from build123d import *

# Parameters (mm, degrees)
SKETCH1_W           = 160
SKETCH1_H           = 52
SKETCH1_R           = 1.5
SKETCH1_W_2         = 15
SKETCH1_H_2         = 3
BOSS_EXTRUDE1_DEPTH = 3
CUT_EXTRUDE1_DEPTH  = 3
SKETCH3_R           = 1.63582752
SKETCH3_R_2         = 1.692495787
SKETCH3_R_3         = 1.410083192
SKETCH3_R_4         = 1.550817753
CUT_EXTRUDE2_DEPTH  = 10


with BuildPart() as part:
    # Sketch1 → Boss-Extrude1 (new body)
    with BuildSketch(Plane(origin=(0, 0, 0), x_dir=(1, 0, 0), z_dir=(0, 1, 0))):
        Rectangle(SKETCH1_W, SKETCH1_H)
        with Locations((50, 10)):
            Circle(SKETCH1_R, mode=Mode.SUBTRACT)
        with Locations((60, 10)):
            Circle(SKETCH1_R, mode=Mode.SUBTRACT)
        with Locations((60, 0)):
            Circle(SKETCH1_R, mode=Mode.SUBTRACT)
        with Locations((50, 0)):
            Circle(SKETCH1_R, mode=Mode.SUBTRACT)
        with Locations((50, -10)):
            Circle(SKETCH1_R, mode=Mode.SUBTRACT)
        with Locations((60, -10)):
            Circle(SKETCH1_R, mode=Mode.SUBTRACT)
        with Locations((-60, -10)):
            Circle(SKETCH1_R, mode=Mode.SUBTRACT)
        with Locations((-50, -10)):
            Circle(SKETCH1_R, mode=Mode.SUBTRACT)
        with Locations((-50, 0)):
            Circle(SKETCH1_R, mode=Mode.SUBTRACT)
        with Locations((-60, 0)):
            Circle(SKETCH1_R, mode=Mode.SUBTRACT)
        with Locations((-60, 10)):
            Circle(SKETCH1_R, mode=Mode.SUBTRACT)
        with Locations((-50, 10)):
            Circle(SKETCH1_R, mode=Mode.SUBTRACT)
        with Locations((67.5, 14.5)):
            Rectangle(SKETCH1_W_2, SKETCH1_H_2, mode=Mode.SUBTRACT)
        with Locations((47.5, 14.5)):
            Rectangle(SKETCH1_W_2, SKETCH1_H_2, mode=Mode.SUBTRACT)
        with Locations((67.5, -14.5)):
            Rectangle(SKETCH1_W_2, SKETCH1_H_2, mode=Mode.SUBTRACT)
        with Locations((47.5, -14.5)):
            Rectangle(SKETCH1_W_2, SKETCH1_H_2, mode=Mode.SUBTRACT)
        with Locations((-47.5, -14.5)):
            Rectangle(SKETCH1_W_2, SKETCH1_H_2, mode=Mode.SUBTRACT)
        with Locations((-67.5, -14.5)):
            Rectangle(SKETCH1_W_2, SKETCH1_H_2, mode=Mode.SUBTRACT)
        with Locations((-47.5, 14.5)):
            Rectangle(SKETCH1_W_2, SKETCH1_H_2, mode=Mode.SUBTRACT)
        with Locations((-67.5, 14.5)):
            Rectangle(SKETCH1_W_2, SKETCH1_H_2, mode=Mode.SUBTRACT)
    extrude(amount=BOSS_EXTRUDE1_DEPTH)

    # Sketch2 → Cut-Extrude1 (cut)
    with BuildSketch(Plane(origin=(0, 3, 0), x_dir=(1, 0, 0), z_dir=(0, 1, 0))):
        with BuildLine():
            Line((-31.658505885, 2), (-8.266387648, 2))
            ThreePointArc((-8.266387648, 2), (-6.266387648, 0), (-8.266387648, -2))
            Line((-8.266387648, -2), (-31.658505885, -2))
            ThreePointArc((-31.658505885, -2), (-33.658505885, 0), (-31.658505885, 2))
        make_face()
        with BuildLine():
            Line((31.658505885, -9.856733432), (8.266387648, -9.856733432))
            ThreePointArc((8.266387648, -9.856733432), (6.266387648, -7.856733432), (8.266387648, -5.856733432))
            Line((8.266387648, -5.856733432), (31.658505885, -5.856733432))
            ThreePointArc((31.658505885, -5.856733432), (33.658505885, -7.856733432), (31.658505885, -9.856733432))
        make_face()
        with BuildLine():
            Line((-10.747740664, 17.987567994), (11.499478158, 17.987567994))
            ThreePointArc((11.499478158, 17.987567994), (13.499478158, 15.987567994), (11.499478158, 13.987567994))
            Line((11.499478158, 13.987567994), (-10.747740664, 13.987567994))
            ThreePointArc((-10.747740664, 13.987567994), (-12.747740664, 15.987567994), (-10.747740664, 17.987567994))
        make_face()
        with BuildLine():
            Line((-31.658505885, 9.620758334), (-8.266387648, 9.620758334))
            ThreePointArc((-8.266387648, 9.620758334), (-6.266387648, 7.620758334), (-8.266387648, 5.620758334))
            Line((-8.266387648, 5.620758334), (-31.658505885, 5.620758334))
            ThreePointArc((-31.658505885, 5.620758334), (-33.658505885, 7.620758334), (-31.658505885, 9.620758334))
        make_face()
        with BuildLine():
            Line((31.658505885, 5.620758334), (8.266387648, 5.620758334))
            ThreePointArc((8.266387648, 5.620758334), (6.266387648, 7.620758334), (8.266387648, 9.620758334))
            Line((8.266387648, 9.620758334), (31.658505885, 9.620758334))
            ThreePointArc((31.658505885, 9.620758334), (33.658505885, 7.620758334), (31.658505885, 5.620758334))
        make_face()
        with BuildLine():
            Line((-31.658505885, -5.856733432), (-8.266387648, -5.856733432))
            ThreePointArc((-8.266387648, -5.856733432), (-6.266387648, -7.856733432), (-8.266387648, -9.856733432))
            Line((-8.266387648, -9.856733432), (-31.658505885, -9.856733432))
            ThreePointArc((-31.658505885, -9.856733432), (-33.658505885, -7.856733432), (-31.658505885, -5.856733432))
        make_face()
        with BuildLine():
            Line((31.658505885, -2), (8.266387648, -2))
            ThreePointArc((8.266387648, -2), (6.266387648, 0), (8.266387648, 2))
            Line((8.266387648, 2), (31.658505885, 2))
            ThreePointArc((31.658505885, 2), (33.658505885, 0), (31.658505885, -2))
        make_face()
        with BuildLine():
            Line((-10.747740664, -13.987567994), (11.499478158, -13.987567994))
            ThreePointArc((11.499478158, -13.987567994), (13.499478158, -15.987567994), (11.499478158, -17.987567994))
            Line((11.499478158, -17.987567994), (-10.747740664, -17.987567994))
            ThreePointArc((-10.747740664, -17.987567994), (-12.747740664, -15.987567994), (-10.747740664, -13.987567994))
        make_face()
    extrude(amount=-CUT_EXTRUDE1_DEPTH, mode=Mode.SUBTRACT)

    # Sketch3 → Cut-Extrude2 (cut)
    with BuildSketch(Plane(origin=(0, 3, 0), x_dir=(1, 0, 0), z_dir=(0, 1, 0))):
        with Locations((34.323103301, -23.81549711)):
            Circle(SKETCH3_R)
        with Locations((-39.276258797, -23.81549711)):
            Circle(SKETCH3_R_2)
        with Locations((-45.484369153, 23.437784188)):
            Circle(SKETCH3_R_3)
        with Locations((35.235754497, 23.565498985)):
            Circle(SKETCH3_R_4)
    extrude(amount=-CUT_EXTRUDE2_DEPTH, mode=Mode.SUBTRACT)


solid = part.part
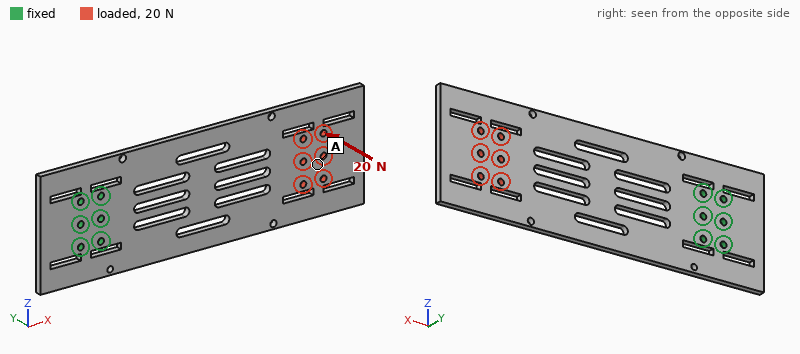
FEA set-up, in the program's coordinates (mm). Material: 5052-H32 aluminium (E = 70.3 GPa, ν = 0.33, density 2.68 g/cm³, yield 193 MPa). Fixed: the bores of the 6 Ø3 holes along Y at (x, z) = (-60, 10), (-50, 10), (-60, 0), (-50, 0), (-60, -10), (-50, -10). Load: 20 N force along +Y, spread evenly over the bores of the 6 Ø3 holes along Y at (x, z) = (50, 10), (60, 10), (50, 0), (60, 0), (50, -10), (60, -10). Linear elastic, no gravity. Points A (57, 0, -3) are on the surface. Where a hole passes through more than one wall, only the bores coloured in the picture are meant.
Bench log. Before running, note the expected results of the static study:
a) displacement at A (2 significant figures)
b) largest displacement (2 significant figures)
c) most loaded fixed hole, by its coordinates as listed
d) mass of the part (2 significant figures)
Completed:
1.2 mm
1.6 mm
(-50, 0)
56 g
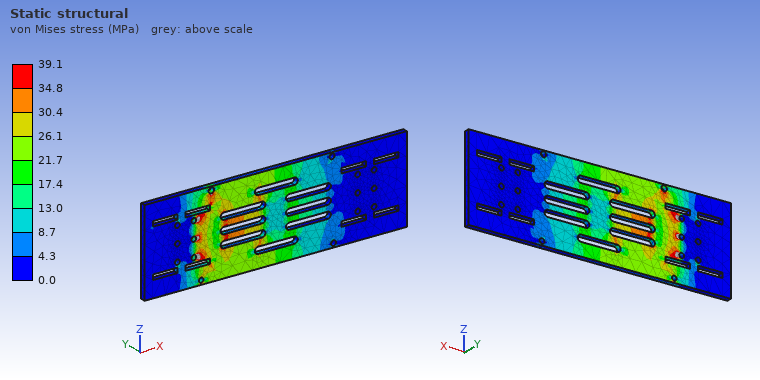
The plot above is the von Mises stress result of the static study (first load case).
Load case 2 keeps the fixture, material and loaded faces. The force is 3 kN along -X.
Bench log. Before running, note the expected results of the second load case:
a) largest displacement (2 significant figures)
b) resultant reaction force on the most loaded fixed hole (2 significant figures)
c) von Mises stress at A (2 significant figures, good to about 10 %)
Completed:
50 µm
820 N
12 MPa
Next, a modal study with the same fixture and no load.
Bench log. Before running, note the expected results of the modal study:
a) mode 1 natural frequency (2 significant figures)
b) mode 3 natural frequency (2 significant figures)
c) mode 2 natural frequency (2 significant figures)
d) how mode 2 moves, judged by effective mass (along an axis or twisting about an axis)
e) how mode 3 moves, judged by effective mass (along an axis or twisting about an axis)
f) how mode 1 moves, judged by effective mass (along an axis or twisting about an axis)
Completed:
140 Hz
880 Hz
610 Hz
twisting about X
along Y
along Y
